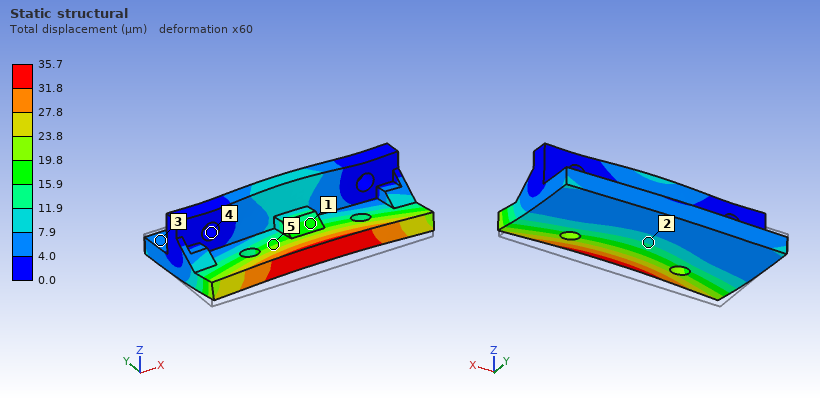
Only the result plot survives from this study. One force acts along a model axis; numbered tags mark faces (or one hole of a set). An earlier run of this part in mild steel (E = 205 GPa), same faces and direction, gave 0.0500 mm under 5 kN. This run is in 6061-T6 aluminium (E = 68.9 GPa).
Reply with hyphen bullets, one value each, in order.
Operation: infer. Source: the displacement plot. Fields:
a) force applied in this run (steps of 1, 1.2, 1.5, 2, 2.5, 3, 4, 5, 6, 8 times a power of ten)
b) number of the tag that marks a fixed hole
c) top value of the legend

- 1.2 kN
- 4
- 35.7 µm
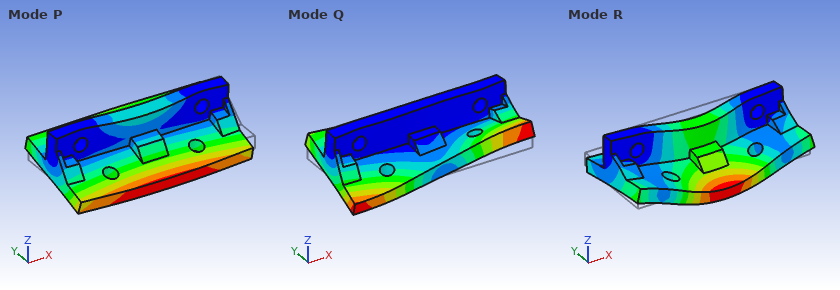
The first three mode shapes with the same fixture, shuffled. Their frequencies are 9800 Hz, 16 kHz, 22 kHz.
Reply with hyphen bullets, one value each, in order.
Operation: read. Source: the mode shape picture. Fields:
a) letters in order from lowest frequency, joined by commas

- P, Q, R
